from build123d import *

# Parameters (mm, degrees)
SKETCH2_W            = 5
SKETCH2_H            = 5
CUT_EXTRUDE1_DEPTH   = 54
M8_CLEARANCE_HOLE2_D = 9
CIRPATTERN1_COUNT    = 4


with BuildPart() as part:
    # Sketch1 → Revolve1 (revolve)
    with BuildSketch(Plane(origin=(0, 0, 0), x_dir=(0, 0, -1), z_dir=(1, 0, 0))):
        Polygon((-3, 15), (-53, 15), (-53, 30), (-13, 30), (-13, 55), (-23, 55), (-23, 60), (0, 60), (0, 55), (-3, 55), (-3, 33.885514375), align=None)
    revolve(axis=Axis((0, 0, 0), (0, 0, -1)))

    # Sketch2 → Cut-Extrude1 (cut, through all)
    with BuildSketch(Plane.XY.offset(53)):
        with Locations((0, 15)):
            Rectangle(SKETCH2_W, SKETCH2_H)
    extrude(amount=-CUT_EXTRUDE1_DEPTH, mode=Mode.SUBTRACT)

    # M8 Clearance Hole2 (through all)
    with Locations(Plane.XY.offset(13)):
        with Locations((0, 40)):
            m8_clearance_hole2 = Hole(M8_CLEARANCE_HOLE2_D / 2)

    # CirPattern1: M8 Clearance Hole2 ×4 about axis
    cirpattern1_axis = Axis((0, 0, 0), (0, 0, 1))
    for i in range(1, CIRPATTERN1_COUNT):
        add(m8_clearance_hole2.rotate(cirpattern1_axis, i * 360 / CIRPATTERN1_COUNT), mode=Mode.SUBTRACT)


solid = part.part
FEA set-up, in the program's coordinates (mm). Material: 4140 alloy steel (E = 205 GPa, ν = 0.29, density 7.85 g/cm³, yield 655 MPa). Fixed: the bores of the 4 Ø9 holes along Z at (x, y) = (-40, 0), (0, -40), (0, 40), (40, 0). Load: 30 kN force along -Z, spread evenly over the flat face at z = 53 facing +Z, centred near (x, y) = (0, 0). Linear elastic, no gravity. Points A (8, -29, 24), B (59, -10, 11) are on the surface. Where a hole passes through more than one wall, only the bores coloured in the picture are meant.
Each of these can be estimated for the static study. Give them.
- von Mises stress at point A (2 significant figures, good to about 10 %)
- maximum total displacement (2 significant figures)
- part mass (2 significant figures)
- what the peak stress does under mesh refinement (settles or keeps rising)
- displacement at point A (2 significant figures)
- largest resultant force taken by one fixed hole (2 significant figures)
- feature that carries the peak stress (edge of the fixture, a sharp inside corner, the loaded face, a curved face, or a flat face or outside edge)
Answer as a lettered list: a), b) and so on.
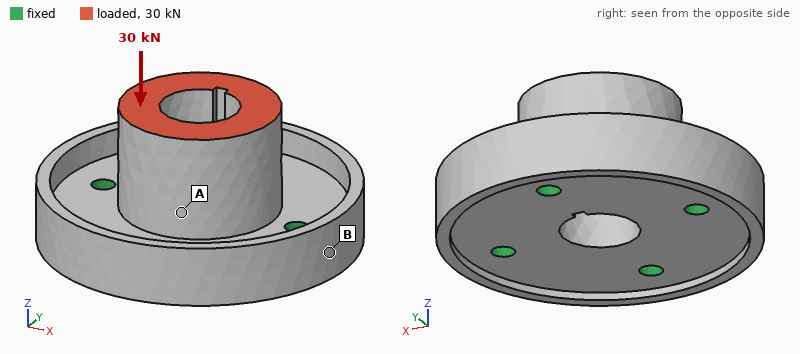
a) 23 MPa
b) 11 µm
c) 1.7 kg
d) keeps rising
e) 8.4 µm
f) 8.0 kN
g) edge of the fixture
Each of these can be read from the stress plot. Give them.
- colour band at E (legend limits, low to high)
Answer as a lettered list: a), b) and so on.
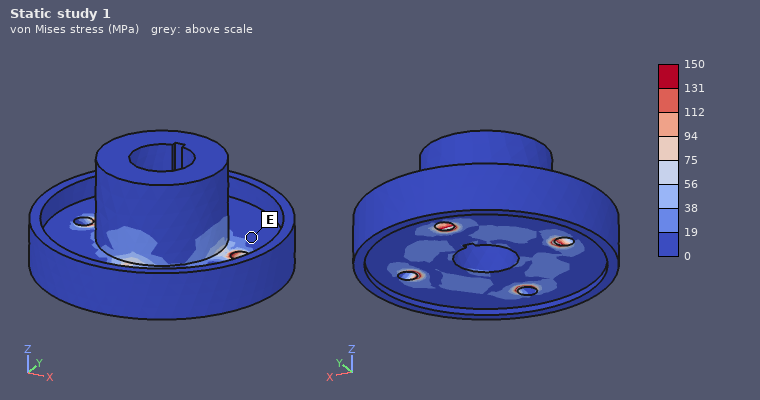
a) 0 to 19 MPa
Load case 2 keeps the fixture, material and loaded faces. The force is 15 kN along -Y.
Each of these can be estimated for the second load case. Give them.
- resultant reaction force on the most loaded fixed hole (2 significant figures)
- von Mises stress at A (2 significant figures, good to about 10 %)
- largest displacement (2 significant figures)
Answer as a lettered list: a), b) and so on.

a) 10 kN
b) 34 MPa
c) 25 µm
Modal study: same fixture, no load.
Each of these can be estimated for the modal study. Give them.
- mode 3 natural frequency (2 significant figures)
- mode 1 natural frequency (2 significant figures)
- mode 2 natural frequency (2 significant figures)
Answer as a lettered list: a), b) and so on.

a) 7300 Hz
b) 6800 Hz
c) 7300 Hz
